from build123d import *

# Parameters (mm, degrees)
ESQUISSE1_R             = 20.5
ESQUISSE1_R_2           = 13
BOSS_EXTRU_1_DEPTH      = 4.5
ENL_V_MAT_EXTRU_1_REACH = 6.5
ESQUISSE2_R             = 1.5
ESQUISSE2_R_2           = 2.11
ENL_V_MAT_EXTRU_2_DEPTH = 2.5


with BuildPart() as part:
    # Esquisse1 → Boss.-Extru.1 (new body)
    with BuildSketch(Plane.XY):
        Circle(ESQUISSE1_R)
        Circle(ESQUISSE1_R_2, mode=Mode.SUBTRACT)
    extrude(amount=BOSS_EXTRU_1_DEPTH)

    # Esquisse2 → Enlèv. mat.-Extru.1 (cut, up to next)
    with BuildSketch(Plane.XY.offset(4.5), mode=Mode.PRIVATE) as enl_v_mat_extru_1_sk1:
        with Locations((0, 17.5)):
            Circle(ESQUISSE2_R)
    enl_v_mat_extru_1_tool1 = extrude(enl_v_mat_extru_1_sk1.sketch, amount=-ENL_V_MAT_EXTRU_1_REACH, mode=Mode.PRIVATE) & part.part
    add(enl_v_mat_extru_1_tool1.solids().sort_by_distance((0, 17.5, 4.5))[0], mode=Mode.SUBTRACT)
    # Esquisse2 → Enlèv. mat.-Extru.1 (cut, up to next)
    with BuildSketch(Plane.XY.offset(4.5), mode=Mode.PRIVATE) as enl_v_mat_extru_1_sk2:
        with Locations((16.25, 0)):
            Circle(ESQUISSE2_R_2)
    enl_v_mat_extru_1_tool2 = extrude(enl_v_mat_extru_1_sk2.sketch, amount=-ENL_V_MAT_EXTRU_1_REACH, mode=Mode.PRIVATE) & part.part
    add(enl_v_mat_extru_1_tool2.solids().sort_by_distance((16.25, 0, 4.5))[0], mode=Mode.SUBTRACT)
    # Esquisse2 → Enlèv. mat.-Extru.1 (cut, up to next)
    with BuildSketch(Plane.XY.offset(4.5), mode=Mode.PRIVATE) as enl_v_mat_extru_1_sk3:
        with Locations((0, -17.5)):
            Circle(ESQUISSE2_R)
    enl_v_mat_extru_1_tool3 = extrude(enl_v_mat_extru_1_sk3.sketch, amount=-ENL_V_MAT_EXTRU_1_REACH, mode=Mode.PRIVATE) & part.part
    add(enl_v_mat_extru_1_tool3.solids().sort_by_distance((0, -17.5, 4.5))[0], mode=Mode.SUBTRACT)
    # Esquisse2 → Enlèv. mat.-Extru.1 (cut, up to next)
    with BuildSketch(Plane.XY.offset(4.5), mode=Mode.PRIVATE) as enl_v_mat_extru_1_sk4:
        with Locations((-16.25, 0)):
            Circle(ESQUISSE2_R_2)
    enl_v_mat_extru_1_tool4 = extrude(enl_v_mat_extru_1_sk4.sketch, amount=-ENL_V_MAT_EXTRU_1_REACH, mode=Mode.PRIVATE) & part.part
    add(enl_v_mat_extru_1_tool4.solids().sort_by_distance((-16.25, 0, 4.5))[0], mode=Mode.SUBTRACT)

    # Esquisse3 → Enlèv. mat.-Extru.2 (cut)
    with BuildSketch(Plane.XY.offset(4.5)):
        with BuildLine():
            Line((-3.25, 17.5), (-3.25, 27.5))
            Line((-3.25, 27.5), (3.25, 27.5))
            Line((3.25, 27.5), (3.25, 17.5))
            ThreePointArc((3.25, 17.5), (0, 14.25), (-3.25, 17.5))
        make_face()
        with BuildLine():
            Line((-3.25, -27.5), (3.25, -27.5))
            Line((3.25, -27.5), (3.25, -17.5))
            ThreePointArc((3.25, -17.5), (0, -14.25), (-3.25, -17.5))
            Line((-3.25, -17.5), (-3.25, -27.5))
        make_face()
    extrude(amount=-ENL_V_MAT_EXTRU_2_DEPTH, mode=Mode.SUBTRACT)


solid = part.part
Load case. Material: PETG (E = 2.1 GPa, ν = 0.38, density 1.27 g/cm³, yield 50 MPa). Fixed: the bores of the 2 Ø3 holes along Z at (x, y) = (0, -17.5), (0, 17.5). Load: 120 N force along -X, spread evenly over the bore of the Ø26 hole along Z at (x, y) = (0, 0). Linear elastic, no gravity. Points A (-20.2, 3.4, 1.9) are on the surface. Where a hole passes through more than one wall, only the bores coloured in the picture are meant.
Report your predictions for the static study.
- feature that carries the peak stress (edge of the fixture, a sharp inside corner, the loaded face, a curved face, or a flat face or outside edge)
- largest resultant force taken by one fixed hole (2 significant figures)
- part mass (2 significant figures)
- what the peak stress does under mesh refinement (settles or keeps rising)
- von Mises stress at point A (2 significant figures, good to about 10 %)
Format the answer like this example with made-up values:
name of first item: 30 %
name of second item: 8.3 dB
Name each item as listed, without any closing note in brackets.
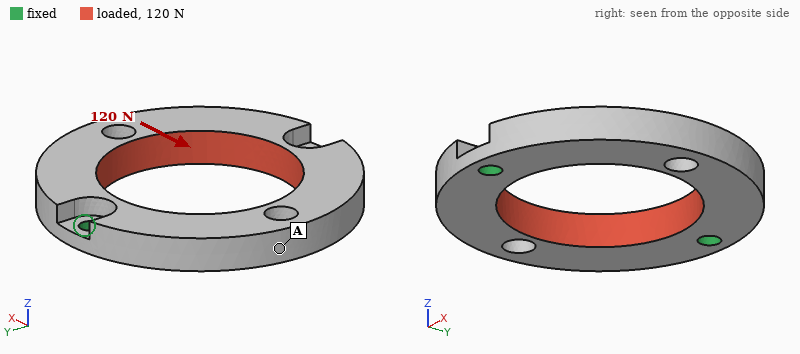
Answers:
feature that carries the peak stress: edge of the fixture
largest resultant force taken by one fixed hole: 60 N
part mass: 4.1 g
what the peak stress does under mesh refinement: keeps rising
von Mises stress at point A: 1.5 MPa
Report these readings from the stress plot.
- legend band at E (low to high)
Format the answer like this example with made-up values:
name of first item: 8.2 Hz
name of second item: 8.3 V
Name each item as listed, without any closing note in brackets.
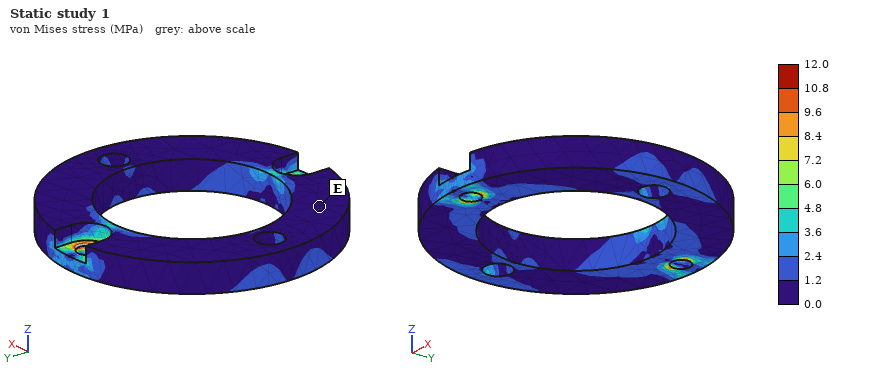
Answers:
legend band at E: 0.0 to 1.2 MPa
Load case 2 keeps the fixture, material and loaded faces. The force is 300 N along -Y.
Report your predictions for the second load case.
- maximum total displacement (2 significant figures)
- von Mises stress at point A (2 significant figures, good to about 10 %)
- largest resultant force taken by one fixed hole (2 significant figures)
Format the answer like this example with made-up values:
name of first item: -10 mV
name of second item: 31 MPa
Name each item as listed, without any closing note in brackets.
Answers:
maximum total displacement: 0.10 mm
von Mises stress at point A: 2.9 MPa
largest resultant force taken by one fixed hole: 150 N
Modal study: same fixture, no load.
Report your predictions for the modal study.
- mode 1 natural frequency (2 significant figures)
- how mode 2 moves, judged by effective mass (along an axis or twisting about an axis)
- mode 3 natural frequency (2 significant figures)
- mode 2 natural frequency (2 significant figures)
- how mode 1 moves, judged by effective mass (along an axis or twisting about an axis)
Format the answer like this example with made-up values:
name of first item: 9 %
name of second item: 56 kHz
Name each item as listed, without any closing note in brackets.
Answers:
mode 1 natural frequency: 870 Hz
how mode 2 moves, judged by effective mass: along Z
mode 3 natural frequency: 3100 Hz
mode 2 natural frequency: 1300 Hz
how mode 1 moves, judged by effective mass: twisting about Y
